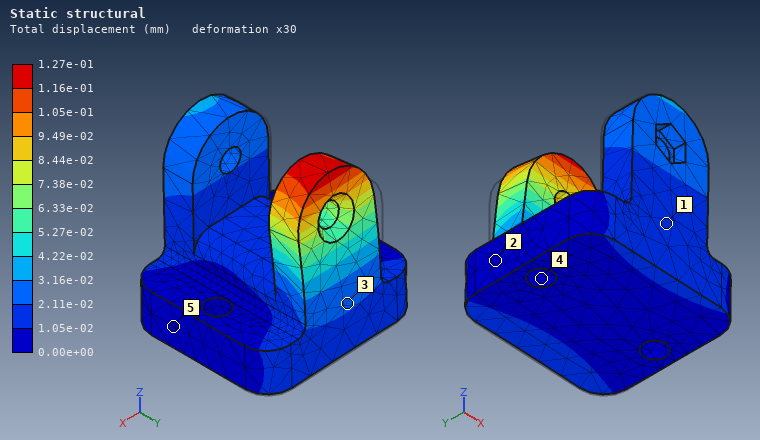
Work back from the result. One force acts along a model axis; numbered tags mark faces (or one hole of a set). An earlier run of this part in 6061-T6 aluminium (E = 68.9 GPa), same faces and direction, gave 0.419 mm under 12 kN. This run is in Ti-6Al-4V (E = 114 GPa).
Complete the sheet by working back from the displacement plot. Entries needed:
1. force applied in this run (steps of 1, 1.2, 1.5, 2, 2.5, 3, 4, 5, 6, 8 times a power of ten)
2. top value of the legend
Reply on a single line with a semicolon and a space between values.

6 kN; 1.27e-01 mm
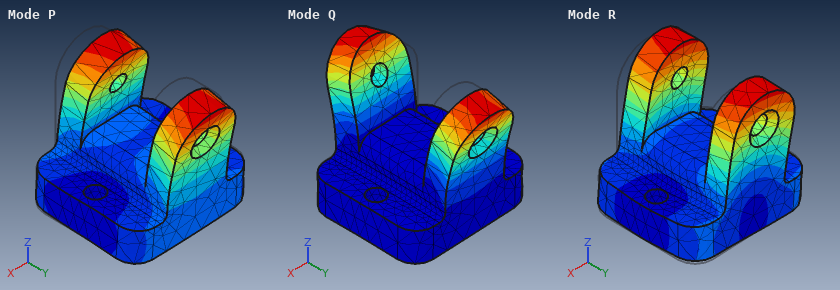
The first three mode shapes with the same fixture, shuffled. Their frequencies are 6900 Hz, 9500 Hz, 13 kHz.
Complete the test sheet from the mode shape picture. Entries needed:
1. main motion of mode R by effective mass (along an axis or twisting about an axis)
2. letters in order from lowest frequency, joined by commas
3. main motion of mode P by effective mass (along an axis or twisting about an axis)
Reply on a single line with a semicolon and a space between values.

along X; P, Q, R; along Y
